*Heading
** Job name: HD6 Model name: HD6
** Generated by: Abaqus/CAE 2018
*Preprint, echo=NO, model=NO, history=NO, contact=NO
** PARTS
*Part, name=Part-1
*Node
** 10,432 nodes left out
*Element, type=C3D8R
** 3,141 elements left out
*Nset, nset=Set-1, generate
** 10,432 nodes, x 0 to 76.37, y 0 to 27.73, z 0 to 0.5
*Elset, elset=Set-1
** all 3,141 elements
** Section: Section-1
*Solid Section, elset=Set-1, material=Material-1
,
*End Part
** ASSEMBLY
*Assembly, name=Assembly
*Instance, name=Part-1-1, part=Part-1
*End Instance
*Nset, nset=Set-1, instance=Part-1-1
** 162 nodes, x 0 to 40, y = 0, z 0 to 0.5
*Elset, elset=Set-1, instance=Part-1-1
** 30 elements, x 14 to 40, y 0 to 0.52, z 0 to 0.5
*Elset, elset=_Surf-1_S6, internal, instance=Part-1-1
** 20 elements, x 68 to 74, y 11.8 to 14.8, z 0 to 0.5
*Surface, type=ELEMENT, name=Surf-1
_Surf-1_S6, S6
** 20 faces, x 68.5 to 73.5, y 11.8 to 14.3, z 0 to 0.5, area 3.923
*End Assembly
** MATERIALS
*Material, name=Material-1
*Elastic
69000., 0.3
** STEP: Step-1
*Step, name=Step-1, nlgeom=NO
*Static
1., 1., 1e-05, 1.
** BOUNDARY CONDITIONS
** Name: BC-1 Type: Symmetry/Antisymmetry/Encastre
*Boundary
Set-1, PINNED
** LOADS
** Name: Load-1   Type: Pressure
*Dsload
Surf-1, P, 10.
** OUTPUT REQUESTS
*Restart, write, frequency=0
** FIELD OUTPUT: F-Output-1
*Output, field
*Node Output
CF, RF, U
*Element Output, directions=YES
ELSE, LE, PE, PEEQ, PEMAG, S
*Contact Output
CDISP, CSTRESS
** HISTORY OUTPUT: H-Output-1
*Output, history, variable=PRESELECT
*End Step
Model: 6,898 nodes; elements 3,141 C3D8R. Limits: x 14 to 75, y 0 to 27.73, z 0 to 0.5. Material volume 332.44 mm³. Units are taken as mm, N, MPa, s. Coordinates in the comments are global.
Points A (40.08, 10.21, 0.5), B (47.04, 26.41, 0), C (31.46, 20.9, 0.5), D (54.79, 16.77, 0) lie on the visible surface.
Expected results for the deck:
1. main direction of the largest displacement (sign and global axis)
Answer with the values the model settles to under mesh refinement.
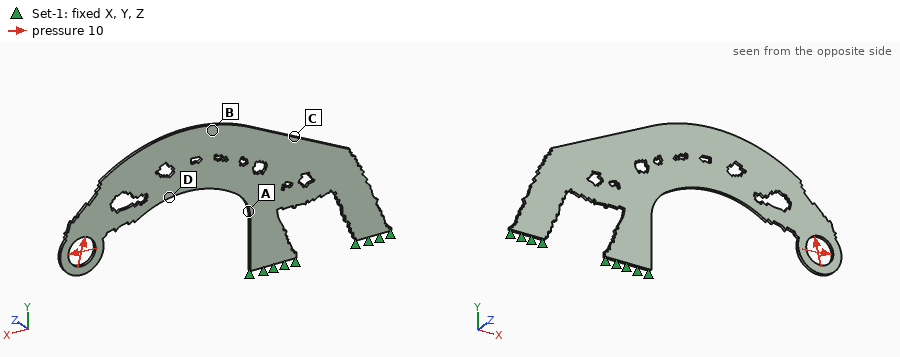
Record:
+Y
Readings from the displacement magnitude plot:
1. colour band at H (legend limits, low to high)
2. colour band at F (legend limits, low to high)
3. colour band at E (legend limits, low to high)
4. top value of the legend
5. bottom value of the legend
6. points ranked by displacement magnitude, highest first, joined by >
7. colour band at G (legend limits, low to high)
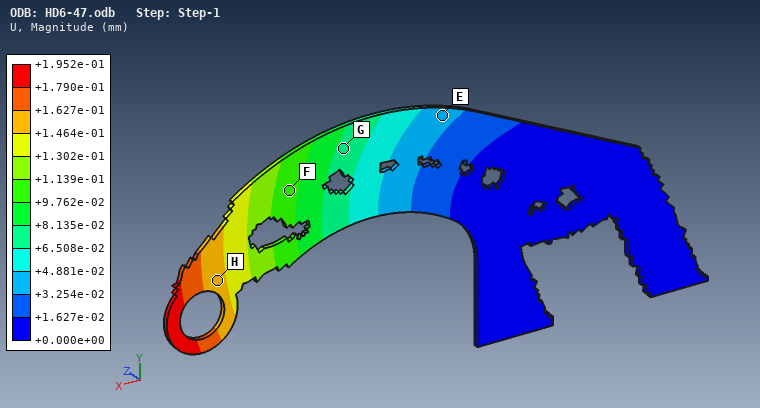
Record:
+1.464e-01 to +1.627e-01 mm
+9.762e-02 to +1.139e-01 mm
+3.254e-02 to +4.881e-02 mm
+1.952e-01 mm
+0.000e+00 mm
H > F > G > E
+6.508e-02 to +8.135e-02 mm
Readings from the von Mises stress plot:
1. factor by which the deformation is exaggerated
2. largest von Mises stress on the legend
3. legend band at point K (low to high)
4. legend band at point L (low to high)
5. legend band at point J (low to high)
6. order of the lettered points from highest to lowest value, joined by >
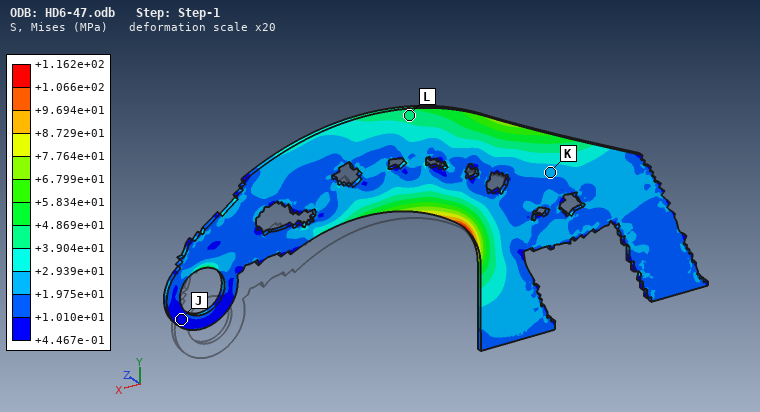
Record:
20
+1.162e+02 MPa
+1.975e+01 to +2.939e+01 MPa
+3.904e+01 to +4.869e+01 MPa
+4.467e-01 to +1.010e+01 MPa
L > K > J
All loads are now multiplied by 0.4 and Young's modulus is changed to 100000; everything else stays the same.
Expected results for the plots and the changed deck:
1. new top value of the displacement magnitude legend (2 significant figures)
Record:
0.054 mm
